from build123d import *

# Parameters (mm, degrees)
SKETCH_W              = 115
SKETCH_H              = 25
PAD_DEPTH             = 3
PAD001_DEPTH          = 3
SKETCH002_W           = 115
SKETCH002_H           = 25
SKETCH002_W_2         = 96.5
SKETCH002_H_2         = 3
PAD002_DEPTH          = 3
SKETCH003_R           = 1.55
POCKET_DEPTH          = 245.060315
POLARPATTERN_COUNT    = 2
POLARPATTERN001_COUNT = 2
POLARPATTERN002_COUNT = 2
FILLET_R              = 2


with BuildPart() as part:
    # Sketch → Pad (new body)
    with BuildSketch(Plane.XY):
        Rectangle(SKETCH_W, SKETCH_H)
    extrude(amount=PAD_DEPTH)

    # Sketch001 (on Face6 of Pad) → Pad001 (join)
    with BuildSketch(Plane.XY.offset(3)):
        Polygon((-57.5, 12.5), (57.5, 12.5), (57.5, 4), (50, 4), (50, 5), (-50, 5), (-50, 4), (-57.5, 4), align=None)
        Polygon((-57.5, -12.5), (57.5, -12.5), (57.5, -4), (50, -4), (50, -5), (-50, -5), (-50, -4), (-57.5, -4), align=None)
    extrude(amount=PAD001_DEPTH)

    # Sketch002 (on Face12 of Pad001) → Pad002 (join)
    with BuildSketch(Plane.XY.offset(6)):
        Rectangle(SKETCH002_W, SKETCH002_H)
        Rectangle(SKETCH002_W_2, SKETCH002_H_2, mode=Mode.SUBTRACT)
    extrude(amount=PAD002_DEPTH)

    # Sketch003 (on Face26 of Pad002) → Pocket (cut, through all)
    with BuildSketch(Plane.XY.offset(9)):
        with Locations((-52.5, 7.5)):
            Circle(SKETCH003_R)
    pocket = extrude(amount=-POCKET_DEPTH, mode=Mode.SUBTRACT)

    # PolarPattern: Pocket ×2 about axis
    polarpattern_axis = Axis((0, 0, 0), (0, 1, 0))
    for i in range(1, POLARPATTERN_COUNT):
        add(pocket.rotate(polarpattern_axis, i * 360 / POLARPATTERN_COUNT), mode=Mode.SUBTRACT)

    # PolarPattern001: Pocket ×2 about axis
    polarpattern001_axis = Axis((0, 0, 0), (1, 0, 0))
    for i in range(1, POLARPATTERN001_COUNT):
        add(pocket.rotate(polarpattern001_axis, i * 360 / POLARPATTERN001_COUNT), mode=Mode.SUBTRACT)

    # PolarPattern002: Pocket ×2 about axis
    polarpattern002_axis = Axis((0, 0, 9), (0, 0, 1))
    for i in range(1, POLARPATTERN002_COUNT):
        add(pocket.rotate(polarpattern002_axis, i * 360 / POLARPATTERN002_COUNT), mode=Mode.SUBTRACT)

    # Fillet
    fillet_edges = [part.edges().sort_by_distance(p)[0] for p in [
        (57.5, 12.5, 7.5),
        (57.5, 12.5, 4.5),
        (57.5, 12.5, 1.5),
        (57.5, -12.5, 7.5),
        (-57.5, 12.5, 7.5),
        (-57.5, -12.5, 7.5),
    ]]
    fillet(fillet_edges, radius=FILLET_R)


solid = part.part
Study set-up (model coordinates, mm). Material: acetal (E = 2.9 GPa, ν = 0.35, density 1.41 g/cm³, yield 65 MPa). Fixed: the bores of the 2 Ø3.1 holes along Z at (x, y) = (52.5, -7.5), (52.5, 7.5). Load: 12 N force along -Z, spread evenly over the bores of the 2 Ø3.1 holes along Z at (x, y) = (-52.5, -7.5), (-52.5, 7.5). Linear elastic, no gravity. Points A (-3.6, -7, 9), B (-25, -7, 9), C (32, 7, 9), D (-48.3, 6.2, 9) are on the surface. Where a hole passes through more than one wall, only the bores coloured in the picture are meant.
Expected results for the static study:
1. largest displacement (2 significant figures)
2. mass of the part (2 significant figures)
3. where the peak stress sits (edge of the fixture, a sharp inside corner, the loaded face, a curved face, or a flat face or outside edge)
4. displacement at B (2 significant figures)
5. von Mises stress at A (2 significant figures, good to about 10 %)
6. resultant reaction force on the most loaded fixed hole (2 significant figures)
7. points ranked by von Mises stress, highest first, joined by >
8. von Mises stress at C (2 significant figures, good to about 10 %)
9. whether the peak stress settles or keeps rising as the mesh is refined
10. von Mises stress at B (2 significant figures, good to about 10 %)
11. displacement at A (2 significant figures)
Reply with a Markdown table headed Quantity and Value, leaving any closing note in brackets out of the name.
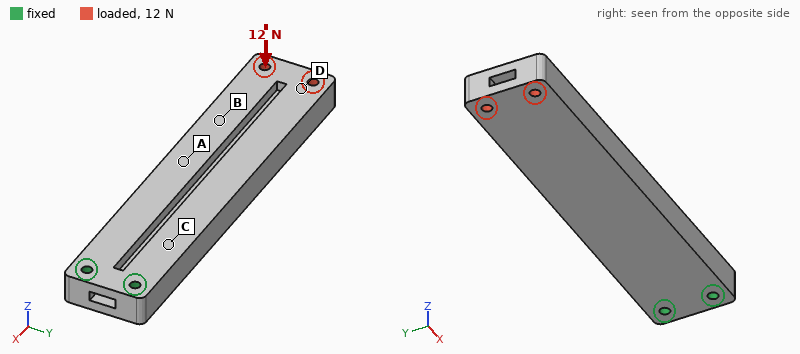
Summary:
| Quantity | Value |
|---|---|
| largest displacement | 1.3 mm |
| mass of the part | 30 g |
| where the peak stress sits | edge of the fixture |
| displacement at B | 0.73 mm |
| von Mises stress at A | 1.9 MPa |
| resultant reaction force on the most loaded fixed hole | 8.6 N |
| points ranked by von Mises stress, highest first, joined by > | C > A > B > D |
| von Mises stress at C | 3.3 MPa |
| whether the peak stress settles or keeps rising as the mesh is refined | keeps rising |
| von Mises stress at B | 1.1 MPa |
| displacement at A | 0.42 mm |
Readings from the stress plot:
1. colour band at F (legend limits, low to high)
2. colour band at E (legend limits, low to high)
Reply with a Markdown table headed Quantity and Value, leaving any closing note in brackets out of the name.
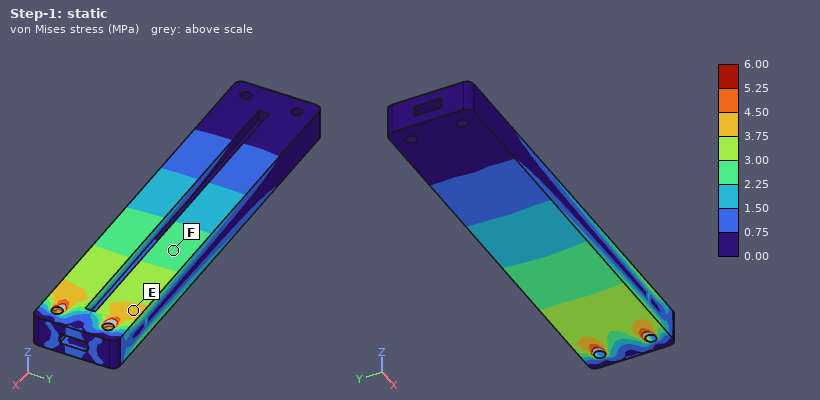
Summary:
| Quantity | Value |
|---|---|
| colour band at F | 2.25 to 3.00 MPa |
| colour band at E | 3.75 to 4.50 MPa |
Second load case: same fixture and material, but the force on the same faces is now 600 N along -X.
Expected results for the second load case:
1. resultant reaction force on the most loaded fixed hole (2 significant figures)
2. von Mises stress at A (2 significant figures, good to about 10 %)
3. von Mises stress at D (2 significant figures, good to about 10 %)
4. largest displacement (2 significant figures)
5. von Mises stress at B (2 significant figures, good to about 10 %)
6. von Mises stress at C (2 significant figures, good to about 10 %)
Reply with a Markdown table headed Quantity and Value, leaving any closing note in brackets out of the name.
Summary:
| Quantity | Value |
|---|---|
| resultant reaction force on the most loaded fixed hole | 300 N |
| von Mises stress at A | 3.5 MPa |
| von Mises stress at D | 3.7 MPa |
| largest displacement | 0.18 mm |
| von Mises stress at B | 3.5 MPa |
| von Mises stress at C | 3.5 MPa |
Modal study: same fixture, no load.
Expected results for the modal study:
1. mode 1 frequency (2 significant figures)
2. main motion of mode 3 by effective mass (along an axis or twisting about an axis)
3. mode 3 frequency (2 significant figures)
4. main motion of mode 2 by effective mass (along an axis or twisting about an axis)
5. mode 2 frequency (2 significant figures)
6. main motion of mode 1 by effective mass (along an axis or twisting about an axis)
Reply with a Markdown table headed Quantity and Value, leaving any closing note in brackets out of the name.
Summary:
| Quantity | Value |
|---|---|
| mode 1 frequency | 180 Hz |
| main motion of mode 3 by effective mass | twisting about X |
| mode 3 frequency | 870 Hz |
| main motion of mode 2 by effective mass | along Y |
| mode 2 frequency | 440 Hz |
| main motion of mode 1 by effective mass | along Z |
